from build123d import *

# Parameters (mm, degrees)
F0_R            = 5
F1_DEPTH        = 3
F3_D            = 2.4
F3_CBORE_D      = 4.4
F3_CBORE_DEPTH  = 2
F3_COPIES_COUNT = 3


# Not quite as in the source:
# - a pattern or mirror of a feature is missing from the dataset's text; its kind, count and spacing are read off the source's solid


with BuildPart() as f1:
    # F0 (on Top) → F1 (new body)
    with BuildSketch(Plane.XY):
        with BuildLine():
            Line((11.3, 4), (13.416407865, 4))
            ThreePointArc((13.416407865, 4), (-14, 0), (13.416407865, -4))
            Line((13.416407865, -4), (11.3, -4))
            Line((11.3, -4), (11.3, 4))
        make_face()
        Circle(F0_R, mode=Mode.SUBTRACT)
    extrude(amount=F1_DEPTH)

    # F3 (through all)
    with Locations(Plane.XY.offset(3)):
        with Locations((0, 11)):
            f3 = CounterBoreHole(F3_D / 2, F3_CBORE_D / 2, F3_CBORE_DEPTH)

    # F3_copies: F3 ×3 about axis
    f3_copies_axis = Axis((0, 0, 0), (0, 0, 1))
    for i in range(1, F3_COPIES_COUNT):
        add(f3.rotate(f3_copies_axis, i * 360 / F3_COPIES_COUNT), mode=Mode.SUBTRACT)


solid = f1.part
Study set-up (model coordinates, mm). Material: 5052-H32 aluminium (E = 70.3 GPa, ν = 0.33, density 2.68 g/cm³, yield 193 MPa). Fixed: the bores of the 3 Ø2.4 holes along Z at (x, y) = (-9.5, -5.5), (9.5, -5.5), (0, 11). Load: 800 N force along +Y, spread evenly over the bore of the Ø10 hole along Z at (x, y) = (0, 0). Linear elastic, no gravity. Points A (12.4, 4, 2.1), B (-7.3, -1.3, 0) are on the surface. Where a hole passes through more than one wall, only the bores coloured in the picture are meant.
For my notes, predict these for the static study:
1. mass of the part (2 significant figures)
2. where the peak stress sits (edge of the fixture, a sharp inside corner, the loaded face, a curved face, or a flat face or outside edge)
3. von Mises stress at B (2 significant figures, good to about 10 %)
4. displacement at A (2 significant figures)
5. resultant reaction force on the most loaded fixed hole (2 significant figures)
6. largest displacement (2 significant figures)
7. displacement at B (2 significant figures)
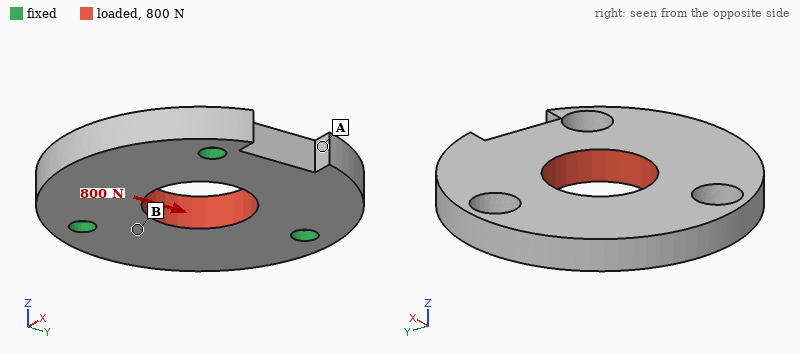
3.9 g
edge of the fixture
20 MPa
4.0 µm
270 N
8.1 µm
2.0 µm
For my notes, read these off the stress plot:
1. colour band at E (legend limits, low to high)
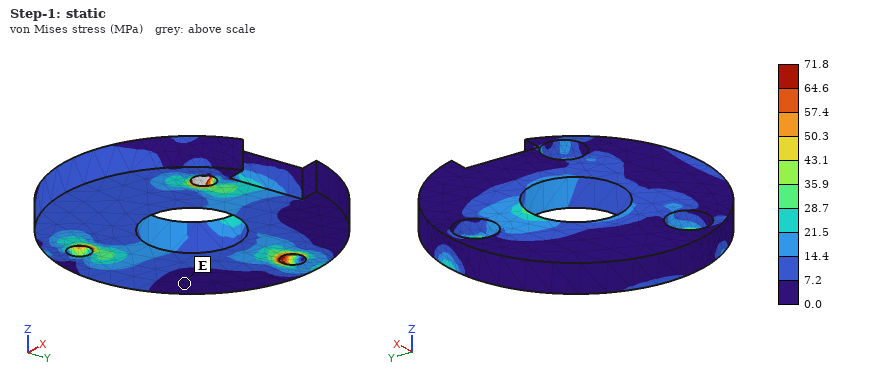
0.0 to 7.2 MPa
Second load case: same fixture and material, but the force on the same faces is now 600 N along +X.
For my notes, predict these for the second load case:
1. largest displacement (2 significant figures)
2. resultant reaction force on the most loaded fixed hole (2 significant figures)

5.2 µm
200 N
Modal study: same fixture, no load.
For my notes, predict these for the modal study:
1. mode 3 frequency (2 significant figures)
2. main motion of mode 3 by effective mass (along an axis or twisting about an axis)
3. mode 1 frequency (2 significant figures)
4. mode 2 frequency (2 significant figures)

23 kHz
along Z
16 kHz
17 kHz
